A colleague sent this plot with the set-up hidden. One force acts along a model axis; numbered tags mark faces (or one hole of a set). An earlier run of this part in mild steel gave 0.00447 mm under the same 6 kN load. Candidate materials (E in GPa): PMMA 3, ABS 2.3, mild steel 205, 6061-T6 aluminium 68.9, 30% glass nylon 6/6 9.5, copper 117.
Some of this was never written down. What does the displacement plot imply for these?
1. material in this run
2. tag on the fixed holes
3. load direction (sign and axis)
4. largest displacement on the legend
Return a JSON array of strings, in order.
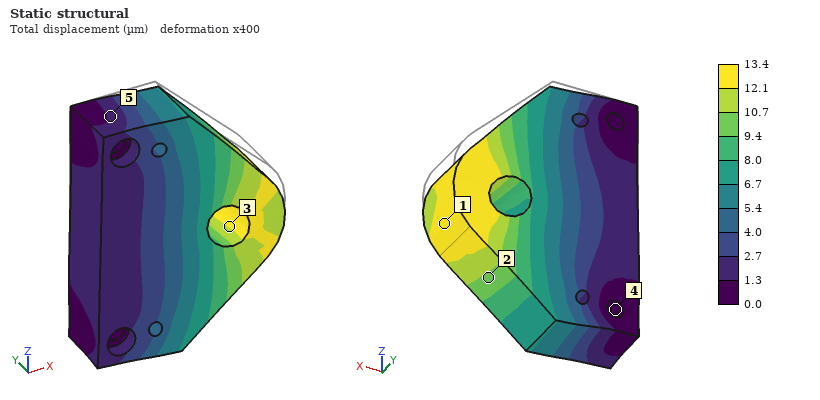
["6061-T6 aluminium", "4", "-Z", "13.4 µm"]
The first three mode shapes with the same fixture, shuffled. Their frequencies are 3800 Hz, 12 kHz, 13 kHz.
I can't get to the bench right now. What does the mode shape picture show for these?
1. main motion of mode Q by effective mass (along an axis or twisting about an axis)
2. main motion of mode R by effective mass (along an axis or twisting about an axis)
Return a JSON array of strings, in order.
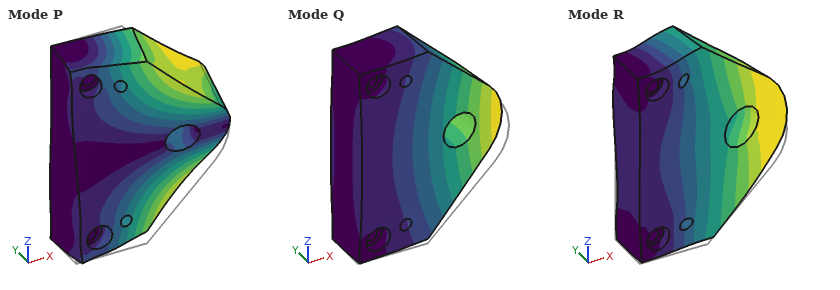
["along Y", "along Z"]
